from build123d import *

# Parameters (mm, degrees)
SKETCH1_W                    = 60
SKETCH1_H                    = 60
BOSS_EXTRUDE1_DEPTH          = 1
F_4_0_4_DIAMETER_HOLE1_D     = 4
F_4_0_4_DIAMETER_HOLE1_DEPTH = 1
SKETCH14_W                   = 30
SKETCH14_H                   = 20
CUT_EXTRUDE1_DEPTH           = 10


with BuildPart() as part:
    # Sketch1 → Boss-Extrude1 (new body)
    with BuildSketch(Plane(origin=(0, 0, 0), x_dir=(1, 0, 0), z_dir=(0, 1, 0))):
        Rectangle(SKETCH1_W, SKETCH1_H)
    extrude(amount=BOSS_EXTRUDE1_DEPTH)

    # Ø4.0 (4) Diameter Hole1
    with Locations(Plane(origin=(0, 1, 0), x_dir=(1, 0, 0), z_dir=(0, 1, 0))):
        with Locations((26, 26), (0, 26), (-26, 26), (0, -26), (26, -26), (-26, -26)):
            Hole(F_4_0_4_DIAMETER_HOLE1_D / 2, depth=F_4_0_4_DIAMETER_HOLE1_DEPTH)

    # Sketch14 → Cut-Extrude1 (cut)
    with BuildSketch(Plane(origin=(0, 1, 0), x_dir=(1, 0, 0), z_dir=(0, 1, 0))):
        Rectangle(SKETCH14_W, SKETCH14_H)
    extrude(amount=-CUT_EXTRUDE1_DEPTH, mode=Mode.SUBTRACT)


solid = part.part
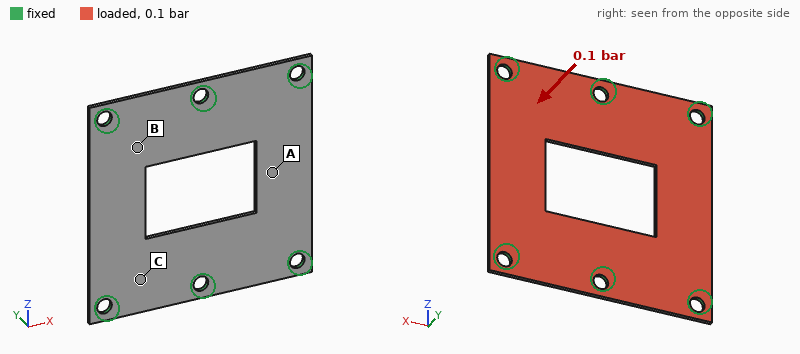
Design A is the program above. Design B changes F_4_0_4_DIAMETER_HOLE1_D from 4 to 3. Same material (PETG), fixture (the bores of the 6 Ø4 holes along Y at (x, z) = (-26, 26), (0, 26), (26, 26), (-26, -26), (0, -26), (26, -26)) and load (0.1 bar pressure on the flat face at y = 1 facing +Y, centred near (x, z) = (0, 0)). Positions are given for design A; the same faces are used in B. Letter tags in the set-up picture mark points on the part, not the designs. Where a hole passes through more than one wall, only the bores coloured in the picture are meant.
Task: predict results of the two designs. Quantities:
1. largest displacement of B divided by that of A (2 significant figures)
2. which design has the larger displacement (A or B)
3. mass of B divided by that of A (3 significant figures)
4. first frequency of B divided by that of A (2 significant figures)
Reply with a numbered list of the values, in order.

1. 1.1
2. B
3. 1.01
4. 0.94
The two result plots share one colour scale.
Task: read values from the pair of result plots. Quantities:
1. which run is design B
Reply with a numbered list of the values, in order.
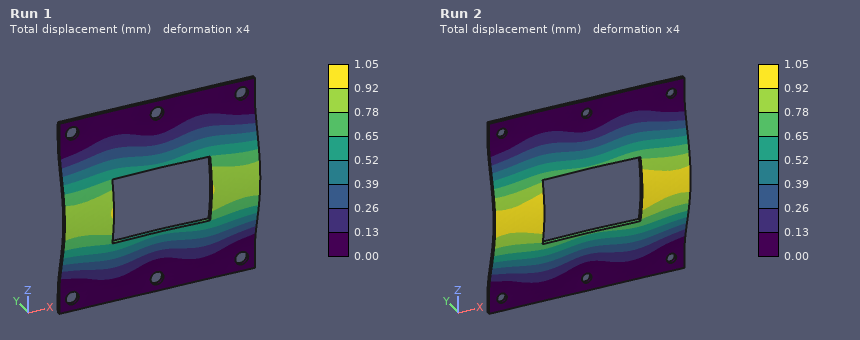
1. Run 2
